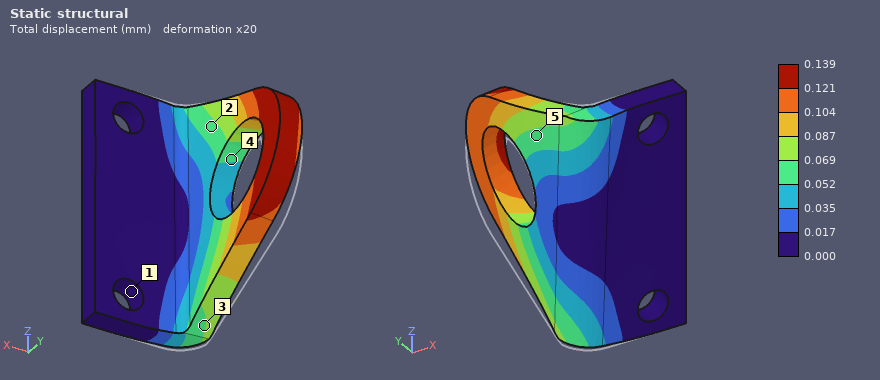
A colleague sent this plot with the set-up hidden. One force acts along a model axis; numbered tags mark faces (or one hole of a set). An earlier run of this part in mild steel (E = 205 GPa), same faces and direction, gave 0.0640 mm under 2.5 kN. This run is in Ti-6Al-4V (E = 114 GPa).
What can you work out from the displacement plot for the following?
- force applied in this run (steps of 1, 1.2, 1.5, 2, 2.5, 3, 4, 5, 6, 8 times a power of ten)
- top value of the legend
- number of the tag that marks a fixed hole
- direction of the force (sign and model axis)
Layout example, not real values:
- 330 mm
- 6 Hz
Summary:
- 3 kN
- 0.139 mm
- 1
- +Z
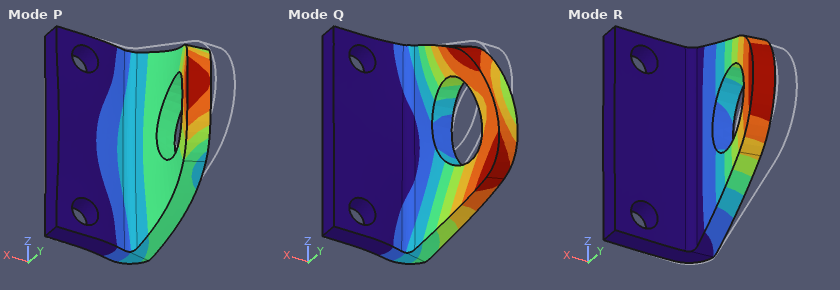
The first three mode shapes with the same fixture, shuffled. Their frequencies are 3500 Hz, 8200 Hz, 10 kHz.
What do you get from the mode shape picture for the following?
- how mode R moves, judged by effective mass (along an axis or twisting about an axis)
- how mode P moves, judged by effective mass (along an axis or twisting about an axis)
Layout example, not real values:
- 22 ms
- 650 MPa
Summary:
- along X
- along Y
